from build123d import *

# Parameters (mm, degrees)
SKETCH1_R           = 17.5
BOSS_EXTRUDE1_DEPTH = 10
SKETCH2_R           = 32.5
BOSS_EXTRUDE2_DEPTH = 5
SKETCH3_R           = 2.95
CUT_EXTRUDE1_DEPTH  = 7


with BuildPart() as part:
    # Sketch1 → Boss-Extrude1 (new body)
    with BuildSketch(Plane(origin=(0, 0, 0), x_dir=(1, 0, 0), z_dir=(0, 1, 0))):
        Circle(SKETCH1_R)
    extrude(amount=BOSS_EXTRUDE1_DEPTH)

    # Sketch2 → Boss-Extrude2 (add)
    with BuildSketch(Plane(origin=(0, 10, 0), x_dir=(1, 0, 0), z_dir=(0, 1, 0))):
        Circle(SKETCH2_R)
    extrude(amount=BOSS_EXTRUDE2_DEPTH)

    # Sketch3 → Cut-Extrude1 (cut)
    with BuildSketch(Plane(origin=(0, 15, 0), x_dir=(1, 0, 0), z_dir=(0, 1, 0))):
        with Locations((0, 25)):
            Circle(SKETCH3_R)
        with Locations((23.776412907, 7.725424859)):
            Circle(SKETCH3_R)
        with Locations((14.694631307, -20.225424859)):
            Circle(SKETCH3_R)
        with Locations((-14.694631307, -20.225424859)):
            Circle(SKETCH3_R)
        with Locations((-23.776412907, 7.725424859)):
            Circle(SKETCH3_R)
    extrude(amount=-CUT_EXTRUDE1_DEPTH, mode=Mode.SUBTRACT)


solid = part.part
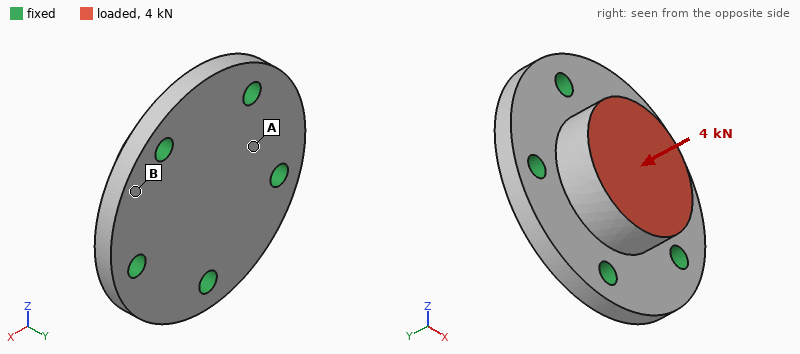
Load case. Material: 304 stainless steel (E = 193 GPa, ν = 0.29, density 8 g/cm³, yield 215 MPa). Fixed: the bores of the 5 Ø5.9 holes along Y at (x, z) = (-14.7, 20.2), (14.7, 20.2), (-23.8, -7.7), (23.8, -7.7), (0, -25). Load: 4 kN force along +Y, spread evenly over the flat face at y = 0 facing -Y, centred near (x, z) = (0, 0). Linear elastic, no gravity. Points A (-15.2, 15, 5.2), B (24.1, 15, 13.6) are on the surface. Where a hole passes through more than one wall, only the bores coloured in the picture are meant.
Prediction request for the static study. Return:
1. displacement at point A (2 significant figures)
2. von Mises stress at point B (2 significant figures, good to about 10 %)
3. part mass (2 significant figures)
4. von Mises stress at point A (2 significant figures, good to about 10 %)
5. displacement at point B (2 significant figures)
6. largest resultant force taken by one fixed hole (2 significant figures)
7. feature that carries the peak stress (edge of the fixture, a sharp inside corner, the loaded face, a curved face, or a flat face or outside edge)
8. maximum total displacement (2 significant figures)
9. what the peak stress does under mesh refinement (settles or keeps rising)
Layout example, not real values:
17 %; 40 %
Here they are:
2.4 µm; 6.7 MPa; 200 g; 13 MPa; 0.57 µm; 870 N; edge of the fixture; 3.1 µm; keeps rising
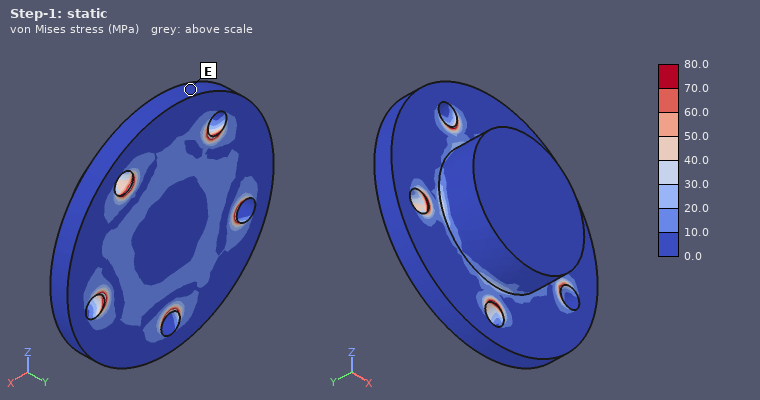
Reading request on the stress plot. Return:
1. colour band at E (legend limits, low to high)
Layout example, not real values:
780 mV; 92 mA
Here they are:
0.0 to 10.0 MPa
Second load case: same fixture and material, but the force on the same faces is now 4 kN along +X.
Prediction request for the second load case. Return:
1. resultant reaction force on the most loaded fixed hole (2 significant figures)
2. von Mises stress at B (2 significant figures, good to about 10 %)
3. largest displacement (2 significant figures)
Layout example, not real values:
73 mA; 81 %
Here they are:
1.4 kN; 9.3 MPa; 4.0 µm
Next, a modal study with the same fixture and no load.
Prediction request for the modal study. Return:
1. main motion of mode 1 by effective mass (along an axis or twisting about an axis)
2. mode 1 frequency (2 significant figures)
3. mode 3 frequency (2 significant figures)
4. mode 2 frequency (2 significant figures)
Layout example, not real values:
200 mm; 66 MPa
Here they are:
along Y; 17 kHz; 21 kHz; 21 kHz
